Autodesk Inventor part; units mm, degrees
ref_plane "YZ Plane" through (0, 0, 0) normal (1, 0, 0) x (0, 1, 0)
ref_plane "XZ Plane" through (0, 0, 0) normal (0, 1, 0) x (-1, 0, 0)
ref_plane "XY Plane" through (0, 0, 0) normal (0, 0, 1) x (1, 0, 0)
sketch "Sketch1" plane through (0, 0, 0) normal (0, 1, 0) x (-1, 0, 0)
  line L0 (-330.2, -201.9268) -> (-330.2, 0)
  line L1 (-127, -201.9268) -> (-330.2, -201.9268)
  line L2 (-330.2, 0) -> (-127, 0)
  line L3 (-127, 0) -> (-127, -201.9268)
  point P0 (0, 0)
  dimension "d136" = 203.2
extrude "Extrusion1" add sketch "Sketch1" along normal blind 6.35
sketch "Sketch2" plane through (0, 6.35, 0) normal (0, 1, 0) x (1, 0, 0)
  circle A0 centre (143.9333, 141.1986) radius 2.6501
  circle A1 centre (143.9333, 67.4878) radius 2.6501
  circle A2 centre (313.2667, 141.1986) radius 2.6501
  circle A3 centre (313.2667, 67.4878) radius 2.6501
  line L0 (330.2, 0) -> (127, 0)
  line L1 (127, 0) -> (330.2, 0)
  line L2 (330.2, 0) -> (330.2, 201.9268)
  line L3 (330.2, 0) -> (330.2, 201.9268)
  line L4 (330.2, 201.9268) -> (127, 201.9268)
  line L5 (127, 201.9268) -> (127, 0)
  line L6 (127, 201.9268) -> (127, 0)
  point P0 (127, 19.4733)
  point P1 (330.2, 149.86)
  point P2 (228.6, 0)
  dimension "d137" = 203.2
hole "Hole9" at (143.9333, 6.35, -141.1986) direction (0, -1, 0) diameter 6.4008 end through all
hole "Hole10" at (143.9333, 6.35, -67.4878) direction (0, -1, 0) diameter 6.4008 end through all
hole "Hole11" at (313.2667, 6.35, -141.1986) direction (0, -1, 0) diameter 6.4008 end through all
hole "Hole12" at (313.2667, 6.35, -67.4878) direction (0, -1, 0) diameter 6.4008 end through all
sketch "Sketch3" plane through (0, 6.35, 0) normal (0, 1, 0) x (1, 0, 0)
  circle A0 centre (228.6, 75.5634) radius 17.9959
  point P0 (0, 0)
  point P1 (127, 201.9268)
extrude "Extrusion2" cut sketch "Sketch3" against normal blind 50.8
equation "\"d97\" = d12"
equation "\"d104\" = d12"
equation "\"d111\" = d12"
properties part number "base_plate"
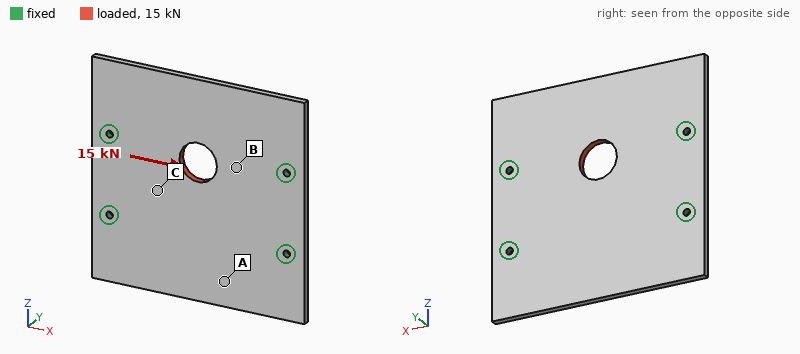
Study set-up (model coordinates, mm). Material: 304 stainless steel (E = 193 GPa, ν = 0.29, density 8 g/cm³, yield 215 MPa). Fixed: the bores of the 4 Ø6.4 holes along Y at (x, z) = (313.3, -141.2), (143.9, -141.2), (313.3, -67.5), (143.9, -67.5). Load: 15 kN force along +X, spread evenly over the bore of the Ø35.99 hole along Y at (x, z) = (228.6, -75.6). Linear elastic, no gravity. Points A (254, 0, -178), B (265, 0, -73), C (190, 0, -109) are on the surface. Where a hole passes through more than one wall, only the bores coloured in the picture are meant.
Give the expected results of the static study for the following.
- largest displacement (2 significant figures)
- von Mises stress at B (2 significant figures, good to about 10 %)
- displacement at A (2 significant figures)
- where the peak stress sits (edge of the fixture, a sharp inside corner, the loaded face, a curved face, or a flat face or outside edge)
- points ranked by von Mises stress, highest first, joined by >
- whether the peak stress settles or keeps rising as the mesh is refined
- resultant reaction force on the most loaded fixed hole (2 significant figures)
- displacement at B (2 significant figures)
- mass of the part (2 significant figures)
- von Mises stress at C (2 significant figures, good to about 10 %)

8.7 µm
20 MPa
1.4 µm
edge of the fixture
B > C > A
keeps rising
5.1 kN
5.5 µm
2.0 kg
10.0 MPa
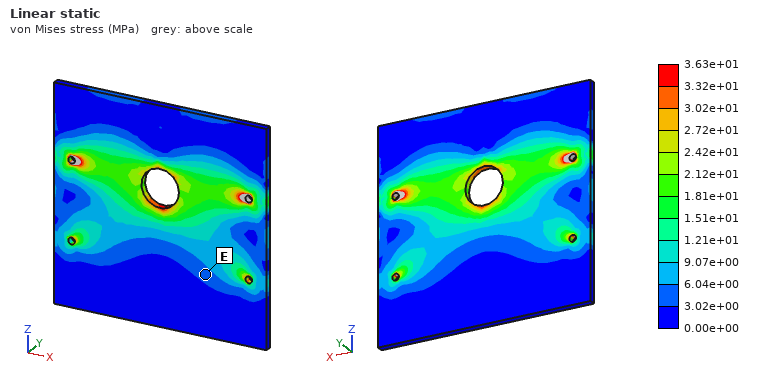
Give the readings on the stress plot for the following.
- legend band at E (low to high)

3.02e+00 to 6.04e+00 MPa
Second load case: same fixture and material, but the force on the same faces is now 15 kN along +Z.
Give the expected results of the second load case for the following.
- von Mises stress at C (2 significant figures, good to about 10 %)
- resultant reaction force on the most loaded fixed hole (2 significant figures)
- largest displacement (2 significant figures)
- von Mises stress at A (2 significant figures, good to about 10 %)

16 MPa
3.9 kN
13 µm
7.0 MPa
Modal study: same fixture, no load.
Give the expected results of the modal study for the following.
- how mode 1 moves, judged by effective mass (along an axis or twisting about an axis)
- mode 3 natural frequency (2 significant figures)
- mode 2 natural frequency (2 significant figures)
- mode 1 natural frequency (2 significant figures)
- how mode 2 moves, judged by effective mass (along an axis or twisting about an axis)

along Y
1200 Hz
780 Hz
690 Hz
along Y
